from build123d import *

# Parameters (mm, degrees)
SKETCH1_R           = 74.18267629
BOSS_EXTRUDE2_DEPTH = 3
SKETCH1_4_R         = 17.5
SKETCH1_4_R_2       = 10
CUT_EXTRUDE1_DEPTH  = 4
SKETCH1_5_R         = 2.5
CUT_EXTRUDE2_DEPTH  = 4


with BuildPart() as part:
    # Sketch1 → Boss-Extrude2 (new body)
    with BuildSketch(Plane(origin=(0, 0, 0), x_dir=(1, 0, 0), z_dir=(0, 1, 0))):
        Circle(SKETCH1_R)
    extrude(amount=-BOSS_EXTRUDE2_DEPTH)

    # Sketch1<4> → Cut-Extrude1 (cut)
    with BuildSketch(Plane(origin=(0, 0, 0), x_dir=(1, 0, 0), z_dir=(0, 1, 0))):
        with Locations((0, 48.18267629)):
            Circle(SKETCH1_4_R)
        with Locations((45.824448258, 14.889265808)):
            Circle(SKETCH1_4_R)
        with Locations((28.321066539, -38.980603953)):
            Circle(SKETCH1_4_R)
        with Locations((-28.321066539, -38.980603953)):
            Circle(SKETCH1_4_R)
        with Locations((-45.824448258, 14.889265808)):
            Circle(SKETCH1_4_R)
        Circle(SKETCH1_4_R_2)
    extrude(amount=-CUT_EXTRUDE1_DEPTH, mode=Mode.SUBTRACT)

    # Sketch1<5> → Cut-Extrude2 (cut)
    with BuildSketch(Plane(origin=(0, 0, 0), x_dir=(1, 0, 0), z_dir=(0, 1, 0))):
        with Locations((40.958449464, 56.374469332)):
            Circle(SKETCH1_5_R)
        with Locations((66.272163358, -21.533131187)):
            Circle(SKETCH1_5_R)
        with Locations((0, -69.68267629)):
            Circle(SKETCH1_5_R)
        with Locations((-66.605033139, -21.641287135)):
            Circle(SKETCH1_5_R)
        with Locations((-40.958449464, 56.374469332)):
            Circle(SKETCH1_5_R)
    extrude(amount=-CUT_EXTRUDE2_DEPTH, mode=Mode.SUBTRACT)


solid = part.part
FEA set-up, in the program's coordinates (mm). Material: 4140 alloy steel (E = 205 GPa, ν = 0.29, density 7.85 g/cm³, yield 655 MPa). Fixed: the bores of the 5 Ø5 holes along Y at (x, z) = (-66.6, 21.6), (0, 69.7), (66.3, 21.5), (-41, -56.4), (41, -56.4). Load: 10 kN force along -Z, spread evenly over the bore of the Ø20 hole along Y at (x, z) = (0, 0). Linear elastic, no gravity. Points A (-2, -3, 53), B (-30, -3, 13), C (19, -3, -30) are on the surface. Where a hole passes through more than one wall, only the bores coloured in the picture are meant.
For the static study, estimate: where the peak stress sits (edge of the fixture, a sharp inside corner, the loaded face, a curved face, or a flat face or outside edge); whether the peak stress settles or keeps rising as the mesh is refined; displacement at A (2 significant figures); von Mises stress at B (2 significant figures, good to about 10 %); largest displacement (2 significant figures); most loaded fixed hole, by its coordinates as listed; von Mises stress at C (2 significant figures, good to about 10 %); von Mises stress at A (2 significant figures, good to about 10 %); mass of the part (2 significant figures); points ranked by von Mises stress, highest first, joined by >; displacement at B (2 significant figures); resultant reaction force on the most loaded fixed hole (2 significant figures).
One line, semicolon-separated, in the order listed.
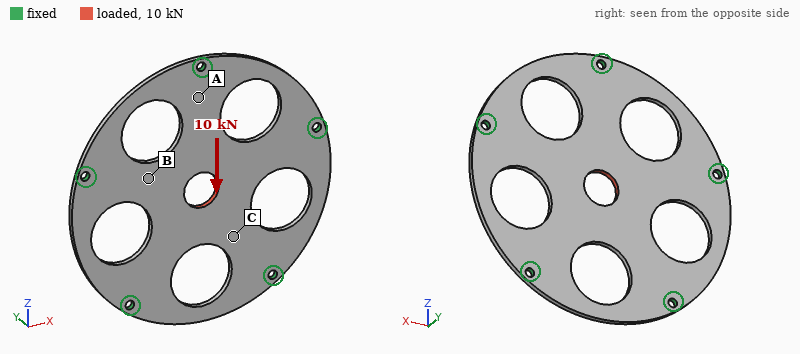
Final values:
edge of the fixture; keeps rising; 5.3 µm; 18 MPa; 16 µm; (0, 69.7); 37 MPa; 56 MPa; 280 g; A > C > B; 10 µm; 3.2 kN
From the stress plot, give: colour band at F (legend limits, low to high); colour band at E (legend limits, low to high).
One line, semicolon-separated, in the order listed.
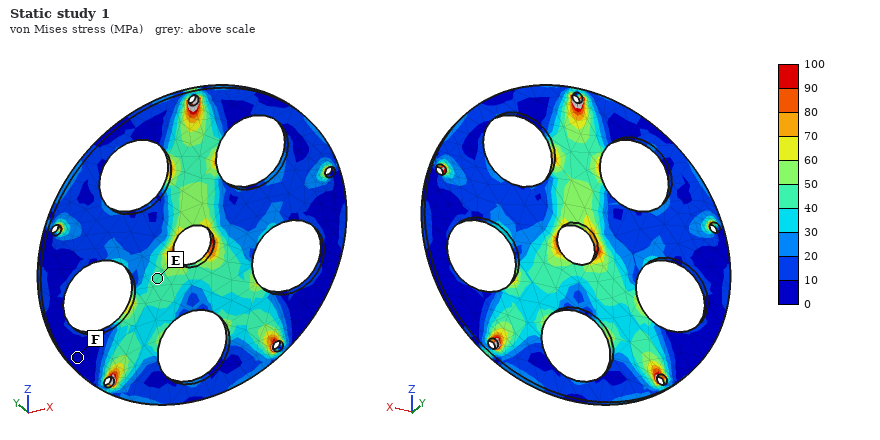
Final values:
0 to 10 MPa; 40 to 50 MPa
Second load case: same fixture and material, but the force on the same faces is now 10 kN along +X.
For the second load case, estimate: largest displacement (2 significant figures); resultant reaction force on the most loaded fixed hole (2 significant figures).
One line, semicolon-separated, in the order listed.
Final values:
16 µm; 3.1 kN
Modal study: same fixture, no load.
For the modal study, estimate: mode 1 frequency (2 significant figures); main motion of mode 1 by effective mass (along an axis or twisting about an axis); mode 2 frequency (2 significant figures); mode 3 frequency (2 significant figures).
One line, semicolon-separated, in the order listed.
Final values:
1200 Hz; along Y; 2400 Hz; 2400 Hz
